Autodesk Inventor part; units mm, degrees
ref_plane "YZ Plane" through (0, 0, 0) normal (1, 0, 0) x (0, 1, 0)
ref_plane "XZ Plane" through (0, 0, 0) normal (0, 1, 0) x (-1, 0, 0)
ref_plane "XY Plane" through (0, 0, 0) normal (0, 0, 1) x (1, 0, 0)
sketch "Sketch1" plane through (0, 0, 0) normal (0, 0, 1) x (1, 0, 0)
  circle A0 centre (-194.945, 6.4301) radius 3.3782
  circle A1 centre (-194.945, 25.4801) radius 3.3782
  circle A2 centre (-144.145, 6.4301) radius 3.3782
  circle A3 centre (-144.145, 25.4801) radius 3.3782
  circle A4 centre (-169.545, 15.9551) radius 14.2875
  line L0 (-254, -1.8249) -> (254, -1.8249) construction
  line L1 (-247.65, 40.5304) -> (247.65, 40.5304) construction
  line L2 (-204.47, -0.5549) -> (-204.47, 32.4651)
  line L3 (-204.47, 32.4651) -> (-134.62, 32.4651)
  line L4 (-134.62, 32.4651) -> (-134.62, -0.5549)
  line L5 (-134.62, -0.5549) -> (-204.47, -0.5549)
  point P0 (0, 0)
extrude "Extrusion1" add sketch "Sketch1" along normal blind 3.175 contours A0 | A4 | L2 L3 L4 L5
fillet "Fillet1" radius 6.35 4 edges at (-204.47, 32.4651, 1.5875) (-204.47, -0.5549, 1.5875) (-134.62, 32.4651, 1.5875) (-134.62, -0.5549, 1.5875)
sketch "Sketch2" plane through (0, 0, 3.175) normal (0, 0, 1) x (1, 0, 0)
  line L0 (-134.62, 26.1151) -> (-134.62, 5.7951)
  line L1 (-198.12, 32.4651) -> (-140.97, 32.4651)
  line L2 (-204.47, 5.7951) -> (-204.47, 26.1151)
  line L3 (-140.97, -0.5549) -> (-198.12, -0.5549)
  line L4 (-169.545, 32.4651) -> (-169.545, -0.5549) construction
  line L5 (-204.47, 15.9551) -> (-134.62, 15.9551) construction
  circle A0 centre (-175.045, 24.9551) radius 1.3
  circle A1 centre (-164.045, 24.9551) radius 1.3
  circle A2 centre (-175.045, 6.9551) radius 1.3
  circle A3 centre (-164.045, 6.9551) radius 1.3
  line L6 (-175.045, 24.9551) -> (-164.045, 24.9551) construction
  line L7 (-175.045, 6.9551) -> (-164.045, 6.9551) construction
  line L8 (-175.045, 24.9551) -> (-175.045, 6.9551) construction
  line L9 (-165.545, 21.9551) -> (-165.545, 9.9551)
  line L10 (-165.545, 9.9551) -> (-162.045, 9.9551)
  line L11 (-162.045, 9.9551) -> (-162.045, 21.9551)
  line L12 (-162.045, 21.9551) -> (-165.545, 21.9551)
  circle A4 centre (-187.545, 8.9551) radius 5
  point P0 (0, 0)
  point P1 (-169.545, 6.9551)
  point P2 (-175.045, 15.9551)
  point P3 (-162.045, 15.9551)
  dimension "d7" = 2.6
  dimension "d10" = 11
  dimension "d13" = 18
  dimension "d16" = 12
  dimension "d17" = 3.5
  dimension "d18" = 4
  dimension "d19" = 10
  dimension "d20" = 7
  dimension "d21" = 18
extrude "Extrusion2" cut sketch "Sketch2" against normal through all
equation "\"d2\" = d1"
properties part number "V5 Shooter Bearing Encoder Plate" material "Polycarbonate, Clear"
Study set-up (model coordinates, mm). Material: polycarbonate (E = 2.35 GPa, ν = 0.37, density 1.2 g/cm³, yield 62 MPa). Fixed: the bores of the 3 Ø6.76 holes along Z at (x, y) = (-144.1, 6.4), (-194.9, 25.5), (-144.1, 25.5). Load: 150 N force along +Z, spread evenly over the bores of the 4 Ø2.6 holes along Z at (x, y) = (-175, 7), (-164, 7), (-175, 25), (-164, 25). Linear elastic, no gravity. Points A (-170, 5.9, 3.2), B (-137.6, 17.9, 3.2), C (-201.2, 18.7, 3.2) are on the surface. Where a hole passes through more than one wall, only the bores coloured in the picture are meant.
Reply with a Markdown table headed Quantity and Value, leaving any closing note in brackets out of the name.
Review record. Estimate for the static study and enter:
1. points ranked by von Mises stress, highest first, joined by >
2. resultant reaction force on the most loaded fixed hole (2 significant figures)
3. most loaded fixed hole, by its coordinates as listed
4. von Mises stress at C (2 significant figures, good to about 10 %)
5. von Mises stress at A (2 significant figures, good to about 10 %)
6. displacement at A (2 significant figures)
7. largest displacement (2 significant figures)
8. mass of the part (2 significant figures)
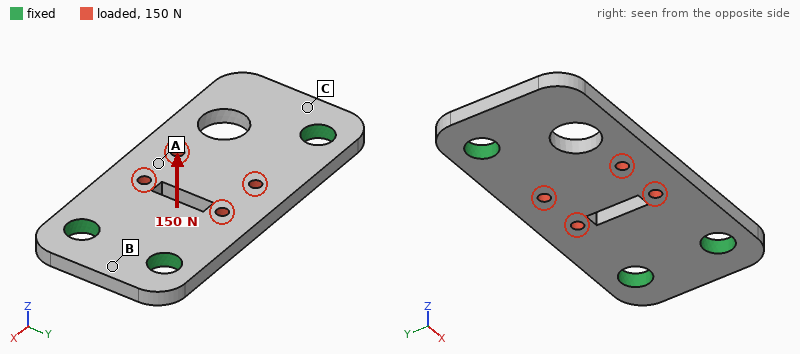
| Quantity | Value |
|---|---|
| points ranked by von Mises stress, highest first, joined by > | A > C > B |
| resultant reaction force on the most loaded fixed hole | 65 N |
| most loaded fixed hole, by its coordinates as listed | (-194.9, 25.5) |
| von Mises stress at C | 5.8 MPa |
| von Mises stress at A | 10.0 MPa |
| displacement at A | 0.61 mm |
| largest displacement | 0.73 mm |
| mass of the part | 7.7 g |
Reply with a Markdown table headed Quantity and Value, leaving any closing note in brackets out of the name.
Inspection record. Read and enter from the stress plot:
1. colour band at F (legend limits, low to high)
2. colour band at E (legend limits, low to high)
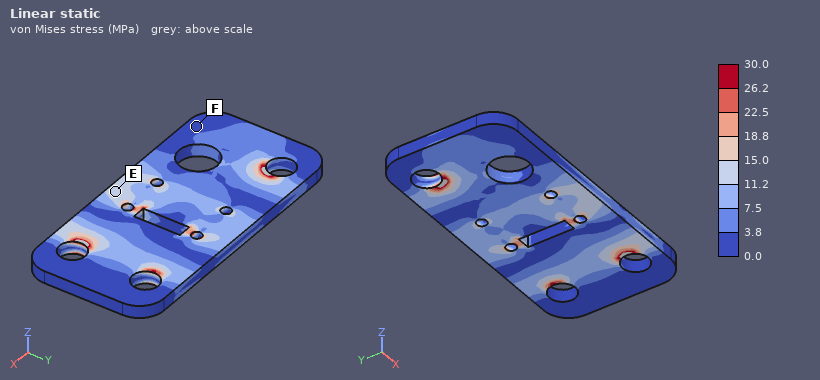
| Quantity | Value |
|---|---|
| colour band at F | 0.0 to 3.8 MPa |
| colour band at E | 11.2 to 15.0 MPa |
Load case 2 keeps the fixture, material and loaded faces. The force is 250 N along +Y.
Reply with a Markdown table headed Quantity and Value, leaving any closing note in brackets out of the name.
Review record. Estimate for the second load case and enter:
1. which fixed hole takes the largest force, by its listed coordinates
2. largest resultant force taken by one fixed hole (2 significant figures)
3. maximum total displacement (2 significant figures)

| Quantity | Value |
|---|---|
| which fixed hole takes the largest force, by its listed coordinates | (-194.9, 25.5) |
| largest resultant force taken by one fixed hole | 120 N |
| maximum total displacement | 61 µm |
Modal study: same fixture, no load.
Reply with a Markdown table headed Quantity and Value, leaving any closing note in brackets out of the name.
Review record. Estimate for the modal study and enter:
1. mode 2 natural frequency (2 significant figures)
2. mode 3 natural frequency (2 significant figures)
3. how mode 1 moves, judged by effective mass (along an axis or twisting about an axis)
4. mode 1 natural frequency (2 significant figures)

| Quantity | Value |
|---|---|
| mode 2 natural frequency | 1900 Hz |
| mode 3 natural frequency | 2600 Hz |
| how mode 1 moves, judged by effective mass | along Z |
| mode 1 natural frequency | 1300 Hz |
